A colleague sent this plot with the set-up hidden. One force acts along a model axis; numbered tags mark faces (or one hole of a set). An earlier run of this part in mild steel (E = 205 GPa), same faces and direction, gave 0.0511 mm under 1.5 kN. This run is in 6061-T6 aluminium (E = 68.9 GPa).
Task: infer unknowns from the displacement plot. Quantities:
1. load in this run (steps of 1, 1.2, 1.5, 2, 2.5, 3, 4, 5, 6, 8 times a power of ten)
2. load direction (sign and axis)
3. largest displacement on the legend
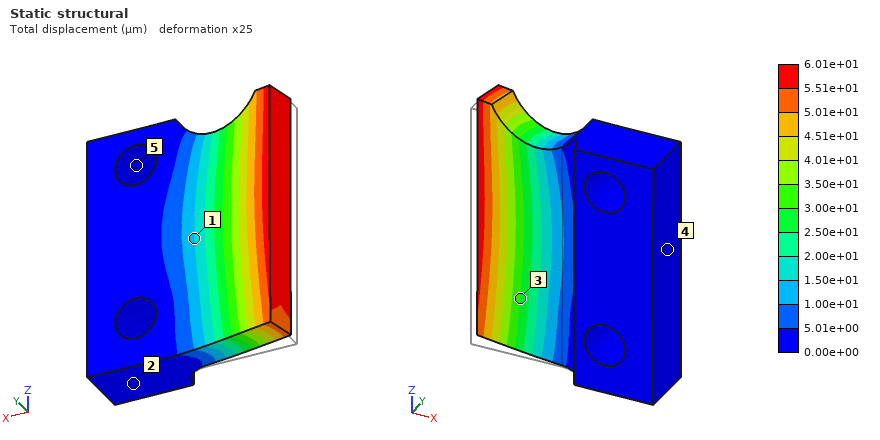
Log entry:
600 N
+Y
6.01e+01 µm
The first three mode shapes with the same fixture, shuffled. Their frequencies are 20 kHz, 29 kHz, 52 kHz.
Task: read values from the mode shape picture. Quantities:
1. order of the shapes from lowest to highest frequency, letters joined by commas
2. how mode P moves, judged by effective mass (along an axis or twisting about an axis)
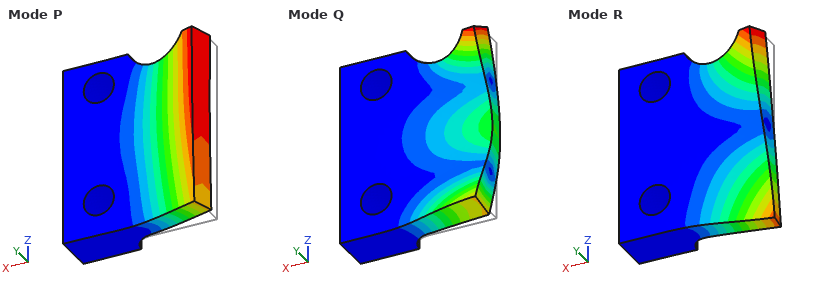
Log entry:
P, R, Q
along Y
